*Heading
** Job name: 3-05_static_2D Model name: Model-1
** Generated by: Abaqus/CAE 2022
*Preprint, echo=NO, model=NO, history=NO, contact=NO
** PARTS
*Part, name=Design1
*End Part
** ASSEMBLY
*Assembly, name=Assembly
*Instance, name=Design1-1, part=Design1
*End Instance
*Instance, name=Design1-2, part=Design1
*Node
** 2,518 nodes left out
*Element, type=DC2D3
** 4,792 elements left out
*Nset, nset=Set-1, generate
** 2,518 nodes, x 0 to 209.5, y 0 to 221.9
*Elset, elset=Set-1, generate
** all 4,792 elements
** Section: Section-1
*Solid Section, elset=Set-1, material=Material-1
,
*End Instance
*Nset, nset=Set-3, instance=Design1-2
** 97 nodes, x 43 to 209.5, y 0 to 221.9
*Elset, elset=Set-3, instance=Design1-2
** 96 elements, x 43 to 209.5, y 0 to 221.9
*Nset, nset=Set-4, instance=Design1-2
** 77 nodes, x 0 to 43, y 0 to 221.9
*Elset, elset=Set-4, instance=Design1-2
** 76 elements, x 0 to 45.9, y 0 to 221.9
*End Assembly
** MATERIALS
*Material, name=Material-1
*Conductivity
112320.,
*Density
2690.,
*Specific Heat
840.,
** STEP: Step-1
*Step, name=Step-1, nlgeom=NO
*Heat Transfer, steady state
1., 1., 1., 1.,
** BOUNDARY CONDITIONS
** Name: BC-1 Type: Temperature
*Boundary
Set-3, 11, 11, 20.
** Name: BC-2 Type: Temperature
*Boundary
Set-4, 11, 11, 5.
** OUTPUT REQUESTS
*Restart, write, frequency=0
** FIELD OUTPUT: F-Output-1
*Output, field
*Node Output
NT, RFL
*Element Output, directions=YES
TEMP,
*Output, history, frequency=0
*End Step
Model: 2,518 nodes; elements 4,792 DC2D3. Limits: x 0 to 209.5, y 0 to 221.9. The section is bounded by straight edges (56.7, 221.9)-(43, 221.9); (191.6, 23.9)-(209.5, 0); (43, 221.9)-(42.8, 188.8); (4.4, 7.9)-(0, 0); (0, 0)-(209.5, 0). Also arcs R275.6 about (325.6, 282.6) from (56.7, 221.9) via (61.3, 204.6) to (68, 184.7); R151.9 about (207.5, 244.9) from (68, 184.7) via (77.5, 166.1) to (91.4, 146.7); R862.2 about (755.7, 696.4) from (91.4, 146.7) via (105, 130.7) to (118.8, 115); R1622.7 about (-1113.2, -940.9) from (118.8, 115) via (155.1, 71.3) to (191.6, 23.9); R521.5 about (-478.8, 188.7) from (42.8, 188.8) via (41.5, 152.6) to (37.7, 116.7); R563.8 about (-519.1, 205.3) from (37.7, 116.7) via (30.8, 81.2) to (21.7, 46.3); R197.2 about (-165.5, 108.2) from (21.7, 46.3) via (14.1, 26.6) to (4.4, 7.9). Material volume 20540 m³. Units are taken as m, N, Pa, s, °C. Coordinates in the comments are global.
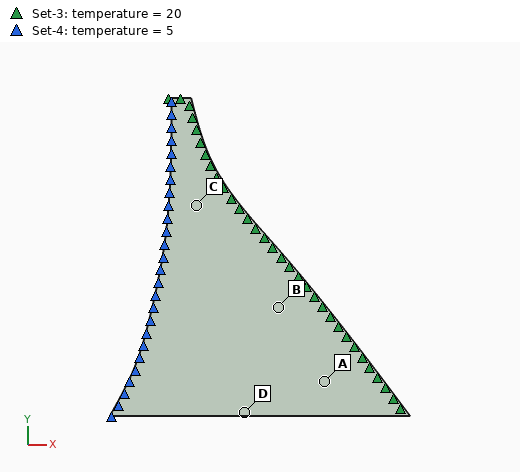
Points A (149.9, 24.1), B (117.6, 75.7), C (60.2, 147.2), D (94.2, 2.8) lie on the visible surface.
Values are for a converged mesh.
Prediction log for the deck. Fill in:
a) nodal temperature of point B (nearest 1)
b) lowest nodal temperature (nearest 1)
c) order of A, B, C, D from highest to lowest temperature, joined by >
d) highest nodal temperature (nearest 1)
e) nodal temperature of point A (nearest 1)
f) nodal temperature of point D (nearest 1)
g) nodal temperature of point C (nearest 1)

17 °C
5 °C
A > B > D > C
20 °C
18 °C
13 °C
11 °C
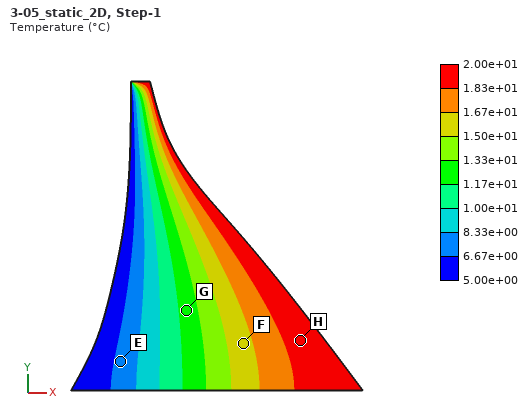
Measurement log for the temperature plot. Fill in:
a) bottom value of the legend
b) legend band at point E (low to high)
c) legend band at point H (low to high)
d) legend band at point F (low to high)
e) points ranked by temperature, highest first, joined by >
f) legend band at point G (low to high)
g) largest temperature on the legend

5.00e+00 °C
6.67e+00 to 8.33e+00 °C
1.83e+01 to 2.00e+01 °C
1.50e+01 to 1.67e+01 °C
H > F > G > E
1.17e+01 to 1.33e+01 °C
2.00e+01 °C
